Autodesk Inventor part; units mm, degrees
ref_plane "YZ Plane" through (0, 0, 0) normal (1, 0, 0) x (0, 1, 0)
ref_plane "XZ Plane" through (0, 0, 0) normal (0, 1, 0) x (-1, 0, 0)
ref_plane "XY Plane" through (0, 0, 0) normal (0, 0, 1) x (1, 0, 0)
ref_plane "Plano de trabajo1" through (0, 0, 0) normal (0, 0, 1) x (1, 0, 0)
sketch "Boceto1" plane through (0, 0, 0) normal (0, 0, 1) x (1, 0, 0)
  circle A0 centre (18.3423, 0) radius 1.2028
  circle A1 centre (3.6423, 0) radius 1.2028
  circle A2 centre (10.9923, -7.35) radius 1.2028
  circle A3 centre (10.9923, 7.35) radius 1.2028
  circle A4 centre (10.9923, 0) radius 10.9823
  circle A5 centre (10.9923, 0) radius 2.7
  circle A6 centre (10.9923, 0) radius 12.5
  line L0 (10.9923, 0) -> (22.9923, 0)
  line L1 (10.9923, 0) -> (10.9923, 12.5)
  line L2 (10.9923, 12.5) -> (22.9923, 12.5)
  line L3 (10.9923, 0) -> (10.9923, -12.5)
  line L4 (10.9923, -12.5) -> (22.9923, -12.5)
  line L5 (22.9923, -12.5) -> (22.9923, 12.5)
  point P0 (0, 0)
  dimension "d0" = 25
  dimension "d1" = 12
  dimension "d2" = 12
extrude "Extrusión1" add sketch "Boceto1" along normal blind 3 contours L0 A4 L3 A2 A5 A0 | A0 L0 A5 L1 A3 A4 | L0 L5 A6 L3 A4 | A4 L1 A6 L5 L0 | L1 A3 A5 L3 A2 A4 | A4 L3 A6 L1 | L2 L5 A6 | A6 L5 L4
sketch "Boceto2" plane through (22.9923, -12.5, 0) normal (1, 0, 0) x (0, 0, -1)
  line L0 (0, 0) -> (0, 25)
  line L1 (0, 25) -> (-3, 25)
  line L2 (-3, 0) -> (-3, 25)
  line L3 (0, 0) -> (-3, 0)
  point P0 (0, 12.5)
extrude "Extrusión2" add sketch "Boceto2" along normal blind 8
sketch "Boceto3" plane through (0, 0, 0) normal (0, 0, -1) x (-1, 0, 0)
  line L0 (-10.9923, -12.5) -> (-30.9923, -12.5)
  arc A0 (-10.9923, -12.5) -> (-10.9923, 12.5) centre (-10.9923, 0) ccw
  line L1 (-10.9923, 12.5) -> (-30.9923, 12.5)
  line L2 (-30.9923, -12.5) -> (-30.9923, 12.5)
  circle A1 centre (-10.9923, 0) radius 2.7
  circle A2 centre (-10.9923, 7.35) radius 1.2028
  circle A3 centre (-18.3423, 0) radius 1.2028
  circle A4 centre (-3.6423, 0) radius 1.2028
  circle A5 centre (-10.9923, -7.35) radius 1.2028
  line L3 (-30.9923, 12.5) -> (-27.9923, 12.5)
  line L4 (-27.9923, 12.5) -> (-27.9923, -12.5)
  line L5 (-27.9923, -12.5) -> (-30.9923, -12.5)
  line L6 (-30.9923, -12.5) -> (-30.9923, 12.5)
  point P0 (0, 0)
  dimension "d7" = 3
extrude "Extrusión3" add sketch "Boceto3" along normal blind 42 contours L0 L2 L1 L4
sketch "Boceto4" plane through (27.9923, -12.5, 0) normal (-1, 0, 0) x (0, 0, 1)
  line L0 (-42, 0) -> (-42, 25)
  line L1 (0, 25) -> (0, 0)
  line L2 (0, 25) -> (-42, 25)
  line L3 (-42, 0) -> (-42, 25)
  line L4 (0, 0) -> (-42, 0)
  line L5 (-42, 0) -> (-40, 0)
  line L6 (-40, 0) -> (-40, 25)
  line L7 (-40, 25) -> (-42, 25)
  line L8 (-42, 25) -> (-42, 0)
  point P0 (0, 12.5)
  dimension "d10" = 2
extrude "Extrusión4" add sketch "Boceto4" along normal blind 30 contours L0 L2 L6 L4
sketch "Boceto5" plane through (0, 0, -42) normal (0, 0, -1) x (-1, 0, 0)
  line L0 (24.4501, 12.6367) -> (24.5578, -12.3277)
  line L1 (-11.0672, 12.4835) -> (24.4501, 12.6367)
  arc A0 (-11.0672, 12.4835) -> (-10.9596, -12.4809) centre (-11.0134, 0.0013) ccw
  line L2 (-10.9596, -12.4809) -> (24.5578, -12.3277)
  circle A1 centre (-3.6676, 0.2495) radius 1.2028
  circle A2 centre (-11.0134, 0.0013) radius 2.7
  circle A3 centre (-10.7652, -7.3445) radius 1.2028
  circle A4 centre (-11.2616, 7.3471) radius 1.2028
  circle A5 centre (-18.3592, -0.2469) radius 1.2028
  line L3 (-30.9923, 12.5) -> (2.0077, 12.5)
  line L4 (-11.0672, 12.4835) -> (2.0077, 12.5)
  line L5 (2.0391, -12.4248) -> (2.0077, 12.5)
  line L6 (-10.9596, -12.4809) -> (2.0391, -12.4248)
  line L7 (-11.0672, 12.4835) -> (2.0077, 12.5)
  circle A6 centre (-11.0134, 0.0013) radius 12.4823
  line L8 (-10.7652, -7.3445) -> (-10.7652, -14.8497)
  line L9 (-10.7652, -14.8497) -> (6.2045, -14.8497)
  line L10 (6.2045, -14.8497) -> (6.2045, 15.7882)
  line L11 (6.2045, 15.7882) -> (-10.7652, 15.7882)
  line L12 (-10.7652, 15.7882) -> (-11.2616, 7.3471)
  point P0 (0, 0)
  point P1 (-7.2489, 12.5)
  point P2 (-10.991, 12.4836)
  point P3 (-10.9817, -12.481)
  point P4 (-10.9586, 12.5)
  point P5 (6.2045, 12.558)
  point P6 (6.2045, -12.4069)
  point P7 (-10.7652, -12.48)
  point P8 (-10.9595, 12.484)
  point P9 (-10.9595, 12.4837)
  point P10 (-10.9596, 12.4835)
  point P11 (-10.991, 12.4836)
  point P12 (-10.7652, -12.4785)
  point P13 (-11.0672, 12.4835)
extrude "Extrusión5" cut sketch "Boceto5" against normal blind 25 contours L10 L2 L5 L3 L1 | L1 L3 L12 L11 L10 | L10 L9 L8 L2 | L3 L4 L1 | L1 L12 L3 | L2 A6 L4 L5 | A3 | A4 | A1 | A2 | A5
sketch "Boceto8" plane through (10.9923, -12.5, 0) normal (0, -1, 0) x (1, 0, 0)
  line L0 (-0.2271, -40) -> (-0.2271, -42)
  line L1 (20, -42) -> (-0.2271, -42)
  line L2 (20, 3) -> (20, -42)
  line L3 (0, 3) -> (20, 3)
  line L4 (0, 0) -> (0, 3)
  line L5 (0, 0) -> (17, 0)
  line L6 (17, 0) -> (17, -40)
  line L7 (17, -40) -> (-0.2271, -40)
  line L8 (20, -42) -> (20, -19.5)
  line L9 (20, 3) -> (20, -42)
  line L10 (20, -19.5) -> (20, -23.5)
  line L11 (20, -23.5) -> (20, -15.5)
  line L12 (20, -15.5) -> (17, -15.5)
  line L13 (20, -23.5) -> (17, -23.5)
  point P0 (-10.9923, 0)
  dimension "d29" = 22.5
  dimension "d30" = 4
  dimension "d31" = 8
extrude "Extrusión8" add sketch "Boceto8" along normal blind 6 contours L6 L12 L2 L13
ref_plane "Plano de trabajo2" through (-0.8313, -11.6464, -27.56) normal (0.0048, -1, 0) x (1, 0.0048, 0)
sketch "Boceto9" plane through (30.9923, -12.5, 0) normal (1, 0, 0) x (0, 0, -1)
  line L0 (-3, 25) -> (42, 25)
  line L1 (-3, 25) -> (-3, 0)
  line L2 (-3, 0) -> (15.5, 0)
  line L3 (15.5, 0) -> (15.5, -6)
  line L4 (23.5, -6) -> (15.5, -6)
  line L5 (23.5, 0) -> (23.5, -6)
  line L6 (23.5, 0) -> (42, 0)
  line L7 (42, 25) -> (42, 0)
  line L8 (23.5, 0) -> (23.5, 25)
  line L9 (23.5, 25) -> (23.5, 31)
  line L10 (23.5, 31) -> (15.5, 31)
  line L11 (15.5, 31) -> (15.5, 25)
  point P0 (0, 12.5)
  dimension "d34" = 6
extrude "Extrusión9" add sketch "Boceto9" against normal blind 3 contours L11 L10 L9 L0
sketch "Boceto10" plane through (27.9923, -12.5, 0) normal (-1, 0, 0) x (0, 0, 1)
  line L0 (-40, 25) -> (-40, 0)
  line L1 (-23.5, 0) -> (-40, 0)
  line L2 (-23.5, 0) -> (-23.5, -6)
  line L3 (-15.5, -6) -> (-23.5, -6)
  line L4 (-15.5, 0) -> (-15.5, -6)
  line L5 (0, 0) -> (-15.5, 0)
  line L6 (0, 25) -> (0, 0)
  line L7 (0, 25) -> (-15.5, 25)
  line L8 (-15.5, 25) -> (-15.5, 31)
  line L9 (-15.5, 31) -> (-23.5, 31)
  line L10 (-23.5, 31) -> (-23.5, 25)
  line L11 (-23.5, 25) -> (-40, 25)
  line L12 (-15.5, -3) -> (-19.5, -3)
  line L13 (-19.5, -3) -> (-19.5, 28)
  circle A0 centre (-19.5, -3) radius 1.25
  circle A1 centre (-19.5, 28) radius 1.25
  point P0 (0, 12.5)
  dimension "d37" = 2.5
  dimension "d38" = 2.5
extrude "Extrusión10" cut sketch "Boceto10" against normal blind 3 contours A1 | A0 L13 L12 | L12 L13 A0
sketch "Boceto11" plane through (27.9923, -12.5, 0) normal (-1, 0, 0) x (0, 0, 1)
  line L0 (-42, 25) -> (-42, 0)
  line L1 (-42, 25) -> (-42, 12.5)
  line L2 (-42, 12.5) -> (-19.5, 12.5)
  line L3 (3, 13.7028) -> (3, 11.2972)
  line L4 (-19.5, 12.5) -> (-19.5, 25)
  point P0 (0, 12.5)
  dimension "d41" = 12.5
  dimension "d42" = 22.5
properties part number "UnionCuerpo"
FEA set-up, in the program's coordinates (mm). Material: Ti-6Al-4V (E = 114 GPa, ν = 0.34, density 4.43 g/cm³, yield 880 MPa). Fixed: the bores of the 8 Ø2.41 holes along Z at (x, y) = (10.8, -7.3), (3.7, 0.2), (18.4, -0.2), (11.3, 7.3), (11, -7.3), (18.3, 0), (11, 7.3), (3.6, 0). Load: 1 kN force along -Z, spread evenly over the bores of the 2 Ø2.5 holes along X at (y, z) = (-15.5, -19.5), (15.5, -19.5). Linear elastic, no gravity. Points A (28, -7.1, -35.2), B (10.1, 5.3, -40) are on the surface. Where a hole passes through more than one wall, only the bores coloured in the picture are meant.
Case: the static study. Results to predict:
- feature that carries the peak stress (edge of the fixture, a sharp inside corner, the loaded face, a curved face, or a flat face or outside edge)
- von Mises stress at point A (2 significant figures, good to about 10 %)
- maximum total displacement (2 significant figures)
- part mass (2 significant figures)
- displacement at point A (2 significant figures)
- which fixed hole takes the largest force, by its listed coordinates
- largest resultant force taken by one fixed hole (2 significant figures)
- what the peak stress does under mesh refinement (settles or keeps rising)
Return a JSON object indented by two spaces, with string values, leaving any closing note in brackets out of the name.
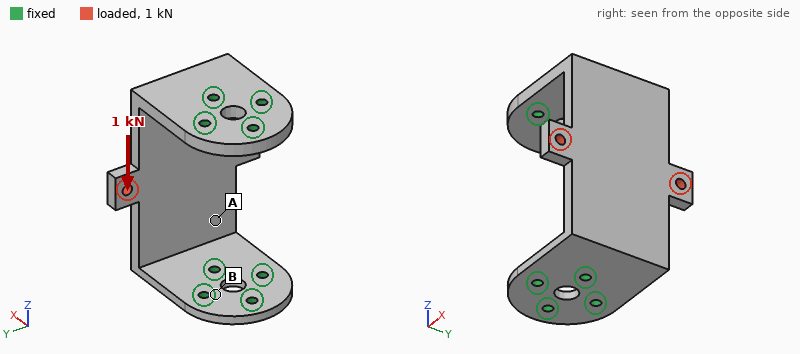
{
  "feature that carries the peak stress": "edge of the fixture",
  "von Mises stress at point A": "42 MPa",
  "maximum total displacement": "48 µm",
  "part mass": "30 g",
  "displacement at point A": "37 µm",
  "which fixed hole takes the largest force, by its listed coordinates": "(18.3, 0)",
  "largest resultant force taken by one fixed hole": "780 N",
  "what the peak stress does under mesh refinement": "keeps rising"
}
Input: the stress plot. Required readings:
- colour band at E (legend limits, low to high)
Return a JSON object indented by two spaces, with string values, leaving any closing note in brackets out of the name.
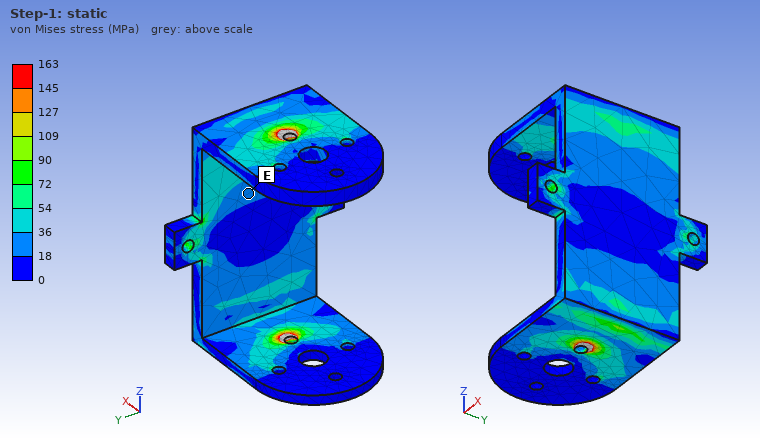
{
  "colour band at E": "18 to 36 MPa"
}
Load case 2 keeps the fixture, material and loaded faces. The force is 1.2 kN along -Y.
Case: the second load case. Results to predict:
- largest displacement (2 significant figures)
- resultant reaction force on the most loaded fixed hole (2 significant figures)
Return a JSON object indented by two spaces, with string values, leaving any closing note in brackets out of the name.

{
  "largest displacement": "16 µm",
  "resultant reaction force on the most loaded fixed hole": "670 N"
}
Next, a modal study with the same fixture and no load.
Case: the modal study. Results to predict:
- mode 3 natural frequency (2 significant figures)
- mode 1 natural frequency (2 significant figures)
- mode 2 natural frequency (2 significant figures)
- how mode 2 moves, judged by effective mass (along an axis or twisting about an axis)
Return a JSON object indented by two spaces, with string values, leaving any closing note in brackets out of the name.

{
  "mode 3 natural frequency": "7700 Hz",
  "mode 1 natural frequency": "5600 Hz",
  "mode 2 natural frequency": "6500 Hz",
  "how mode 2 moves, judged by effective mass": "along Z"
}
